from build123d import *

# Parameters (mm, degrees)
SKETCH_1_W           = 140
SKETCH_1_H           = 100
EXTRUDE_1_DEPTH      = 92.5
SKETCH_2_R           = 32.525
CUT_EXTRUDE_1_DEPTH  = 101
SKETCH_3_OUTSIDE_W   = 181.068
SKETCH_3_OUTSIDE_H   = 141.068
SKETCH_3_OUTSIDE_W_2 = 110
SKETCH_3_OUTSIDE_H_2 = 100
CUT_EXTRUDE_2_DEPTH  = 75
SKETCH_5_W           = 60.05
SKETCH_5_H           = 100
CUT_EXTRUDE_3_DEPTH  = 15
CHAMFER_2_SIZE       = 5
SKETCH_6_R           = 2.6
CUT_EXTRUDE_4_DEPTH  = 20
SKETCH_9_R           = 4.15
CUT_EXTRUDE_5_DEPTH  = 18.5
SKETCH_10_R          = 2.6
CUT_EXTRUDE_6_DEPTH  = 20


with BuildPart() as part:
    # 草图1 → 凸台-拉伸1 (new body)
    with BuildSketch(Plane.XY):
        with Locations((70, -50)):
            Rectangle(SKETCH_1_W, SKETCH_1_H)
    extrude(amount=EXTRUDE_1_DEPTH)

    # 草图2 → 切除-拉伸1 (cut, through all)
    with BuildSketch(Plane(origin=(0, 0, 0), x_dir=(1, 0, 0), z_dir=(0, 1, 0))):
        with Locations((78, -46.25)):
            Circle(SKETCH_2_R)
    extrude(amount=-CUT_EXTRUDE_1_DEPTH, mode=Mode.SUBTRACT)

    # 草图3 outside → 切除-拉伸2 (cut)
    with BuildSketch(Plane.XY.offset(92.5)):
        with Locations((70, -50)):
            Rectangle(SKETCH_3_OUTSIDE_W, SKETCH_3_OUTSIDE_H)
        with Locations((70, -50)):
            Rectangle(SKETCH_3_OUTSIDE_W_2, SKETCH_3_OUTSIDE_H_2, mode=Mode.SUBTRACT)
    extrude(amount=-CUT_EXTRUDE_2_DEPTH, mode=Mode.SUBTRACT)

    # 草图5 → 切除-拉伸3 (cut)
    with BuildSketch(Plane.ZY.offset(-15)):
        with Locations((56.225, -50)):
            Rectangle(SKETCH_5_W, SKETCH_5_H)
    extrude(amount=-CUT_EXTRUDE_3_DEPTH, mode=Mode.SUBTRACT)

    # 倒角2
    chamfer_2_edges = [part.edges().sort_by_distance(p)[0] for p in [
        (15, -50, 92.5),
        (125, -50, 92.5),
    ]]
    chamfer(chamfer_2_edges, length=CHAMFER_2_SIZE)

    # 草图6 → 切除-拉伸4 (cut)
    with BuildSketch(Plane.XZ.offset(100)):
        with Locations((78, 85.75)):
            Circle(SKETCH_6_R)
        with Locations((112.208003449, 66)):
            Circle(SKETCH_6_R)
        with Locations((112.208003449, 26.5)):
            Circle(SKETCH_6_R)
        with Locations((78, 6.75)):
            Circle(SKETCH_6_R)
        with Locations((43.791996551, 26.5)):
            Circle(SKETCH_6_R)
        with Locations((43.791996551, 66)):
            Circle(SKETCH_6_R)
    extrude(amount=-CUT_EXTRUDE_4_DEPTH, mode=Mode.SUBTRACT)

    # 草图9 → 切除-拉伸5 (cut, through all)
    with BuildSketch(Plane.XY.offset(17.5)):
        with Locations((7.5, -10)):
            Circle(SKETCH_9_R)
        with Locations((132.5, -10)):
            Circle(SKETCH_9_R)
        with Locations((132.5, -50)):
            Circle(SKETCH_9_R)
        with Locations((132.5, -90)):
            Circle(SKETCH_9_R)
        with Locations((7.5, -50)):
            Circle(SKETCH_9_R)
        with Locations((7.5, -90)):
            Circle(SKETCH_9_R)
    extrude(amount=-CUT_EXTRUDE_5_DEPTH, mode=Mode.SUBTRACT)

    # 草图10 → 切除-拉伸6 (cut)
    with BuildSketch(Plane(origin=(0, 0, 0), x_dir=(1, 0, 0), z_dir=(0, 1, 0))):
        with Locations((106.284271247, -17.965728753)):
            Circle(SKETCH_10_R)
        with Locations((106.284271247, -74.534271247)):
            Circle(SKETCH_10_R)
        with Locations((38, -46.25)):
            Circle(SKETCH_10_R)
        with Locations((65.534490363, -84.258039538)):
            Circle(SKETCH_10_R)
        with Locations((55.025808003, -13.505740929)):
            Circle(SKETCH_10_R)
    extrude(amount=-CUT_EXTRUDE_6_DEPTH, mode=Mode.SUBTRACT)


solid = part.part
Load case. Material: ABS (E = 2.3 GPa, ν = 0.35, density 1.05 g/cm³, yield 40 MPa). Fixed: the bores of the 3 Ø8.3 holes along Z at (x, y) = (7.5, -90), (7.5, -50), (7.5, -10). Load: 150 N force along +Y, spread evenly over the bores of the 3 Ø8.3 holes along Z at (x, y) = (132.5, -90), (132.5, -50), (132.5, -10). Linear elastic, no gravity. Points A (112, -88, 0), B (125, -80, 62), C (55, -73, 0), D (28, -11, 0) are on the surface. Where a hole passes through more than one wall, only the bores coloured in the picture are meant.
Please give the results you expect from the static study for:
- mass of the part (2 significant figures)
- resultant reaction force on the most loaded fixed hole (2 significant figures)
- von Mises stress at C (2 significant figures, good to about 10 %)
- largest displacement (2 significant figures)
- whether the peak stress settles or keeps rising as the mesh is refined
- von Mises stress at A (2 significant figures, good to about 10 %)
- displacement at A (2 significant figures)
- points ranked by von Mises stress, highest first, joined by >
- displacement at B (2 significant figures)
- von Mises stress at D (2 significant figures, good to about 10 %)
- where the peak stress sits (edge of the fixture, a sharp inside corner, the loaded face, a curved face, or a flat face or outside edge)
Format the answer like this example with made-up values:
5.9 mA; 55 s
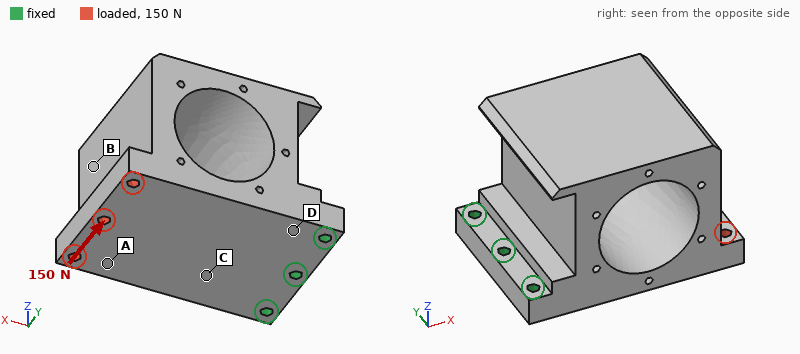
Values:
670 g; 230 N; 0.26 MPa; 51 µm; keeps rising; 0.14 MPa; 37 µm; D > C > A > B; 32 µm; 0.47 MPa; edge of the fixture
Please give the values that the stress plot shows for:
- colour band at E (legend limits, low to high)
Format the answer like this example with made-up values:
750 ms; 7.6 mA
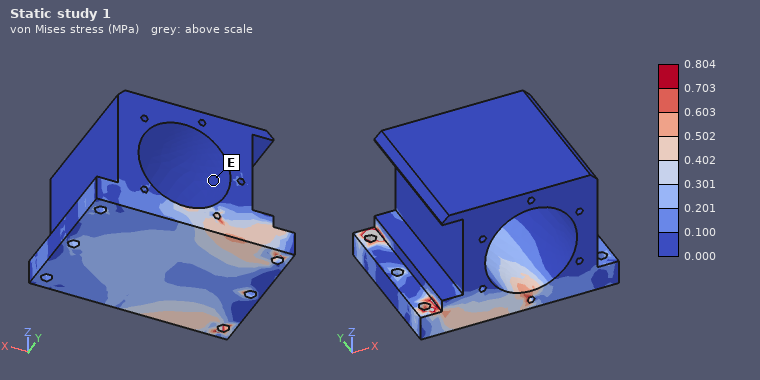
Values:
0.000 to 0.100 MPa
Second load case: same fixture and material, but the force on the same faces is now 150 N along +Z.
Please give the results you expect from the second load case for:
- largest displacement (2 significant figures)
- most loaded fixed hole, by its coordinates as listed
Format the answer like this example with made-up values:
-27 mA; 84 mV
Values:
0.56 mm; (7.5, -50)
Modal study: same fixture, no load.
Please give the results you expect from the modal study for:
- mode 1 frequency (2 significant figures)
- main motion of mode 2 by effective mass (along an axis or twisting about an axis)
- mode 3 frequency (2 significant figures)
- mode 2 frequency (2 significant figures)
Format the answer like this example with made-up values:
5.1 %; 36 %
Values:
160 Hz; along Y; 750 Hz; 500 Hz
